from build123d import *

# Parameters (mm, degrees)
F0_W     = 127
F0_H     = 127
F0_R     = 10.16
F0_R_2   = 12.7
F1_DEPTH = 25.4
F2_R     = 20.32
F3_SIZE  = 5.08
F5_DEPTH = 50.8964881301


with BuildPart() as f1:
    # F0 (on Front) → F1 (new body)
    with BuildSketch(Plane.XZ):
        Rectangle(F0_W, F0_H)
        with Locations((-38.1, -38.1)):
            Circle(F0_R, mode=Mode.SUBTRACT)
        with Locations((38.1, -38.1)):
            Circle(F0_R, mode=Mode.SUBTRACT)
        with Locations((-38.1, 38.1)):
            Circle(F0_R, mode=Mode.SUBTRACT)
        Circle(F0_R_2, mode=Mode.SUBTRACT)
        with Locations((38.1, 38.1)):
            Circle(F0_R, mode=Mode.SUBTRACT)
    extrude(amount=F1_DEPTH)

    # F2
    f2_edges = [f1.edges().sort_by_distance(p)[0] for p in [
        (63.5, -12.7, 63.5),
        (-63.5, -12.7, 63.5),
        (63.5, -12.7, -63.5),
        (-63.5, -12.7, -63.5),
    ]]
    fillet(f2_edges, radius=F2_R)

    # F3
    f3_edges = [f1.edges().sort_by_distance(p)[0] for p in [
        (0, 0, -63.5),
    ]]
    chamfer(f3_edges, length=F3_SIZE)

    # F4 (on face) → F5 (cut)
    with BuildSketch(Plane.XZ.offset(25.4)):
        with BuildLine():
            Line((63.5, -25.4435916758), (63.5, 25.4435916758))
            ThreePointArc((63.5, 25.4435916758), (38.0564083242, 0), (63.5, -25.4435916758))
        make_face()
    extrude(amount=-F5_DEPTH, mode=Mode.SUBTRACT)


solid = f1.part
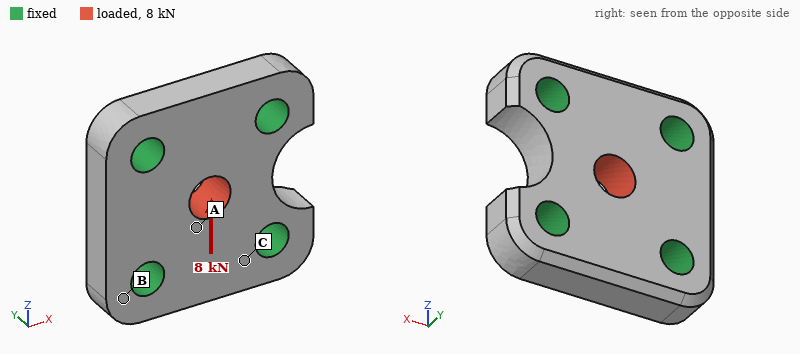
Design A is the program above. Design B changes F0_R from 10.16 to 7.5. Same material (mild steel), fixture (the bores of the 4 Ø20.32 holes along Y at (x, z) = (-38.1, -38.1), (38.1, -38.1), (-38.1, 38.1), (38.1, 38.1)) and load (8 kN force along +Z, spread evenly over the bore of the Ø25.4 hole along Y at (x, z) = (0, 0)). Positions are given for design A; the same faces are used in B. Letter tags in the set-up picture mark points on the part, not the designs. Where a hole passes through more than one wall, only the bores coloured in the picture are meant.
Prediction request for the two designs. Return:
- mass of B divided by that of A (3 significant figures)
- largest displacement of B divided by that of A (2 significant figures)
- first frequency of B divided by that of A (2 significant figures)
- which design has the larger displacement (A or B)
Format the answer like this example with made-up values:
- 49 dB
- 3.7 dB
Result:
- 1.05
- 1.1
- 0.87
- B
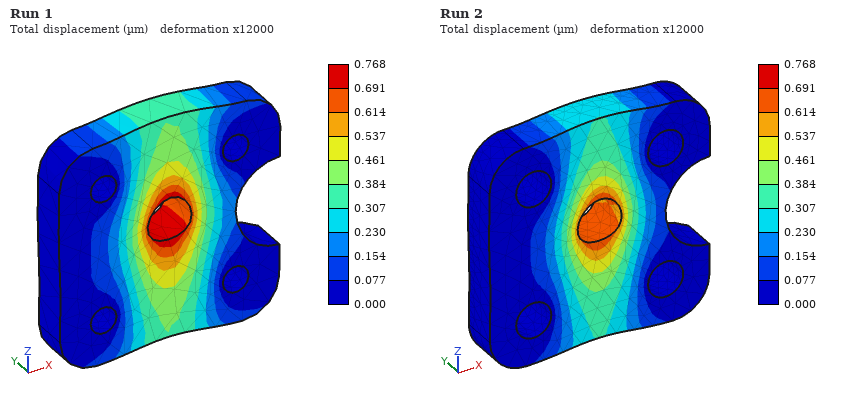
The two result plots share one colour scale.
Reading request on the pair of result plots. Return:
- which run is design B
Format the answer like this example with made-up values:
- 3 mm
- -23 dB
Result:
- Run 1
